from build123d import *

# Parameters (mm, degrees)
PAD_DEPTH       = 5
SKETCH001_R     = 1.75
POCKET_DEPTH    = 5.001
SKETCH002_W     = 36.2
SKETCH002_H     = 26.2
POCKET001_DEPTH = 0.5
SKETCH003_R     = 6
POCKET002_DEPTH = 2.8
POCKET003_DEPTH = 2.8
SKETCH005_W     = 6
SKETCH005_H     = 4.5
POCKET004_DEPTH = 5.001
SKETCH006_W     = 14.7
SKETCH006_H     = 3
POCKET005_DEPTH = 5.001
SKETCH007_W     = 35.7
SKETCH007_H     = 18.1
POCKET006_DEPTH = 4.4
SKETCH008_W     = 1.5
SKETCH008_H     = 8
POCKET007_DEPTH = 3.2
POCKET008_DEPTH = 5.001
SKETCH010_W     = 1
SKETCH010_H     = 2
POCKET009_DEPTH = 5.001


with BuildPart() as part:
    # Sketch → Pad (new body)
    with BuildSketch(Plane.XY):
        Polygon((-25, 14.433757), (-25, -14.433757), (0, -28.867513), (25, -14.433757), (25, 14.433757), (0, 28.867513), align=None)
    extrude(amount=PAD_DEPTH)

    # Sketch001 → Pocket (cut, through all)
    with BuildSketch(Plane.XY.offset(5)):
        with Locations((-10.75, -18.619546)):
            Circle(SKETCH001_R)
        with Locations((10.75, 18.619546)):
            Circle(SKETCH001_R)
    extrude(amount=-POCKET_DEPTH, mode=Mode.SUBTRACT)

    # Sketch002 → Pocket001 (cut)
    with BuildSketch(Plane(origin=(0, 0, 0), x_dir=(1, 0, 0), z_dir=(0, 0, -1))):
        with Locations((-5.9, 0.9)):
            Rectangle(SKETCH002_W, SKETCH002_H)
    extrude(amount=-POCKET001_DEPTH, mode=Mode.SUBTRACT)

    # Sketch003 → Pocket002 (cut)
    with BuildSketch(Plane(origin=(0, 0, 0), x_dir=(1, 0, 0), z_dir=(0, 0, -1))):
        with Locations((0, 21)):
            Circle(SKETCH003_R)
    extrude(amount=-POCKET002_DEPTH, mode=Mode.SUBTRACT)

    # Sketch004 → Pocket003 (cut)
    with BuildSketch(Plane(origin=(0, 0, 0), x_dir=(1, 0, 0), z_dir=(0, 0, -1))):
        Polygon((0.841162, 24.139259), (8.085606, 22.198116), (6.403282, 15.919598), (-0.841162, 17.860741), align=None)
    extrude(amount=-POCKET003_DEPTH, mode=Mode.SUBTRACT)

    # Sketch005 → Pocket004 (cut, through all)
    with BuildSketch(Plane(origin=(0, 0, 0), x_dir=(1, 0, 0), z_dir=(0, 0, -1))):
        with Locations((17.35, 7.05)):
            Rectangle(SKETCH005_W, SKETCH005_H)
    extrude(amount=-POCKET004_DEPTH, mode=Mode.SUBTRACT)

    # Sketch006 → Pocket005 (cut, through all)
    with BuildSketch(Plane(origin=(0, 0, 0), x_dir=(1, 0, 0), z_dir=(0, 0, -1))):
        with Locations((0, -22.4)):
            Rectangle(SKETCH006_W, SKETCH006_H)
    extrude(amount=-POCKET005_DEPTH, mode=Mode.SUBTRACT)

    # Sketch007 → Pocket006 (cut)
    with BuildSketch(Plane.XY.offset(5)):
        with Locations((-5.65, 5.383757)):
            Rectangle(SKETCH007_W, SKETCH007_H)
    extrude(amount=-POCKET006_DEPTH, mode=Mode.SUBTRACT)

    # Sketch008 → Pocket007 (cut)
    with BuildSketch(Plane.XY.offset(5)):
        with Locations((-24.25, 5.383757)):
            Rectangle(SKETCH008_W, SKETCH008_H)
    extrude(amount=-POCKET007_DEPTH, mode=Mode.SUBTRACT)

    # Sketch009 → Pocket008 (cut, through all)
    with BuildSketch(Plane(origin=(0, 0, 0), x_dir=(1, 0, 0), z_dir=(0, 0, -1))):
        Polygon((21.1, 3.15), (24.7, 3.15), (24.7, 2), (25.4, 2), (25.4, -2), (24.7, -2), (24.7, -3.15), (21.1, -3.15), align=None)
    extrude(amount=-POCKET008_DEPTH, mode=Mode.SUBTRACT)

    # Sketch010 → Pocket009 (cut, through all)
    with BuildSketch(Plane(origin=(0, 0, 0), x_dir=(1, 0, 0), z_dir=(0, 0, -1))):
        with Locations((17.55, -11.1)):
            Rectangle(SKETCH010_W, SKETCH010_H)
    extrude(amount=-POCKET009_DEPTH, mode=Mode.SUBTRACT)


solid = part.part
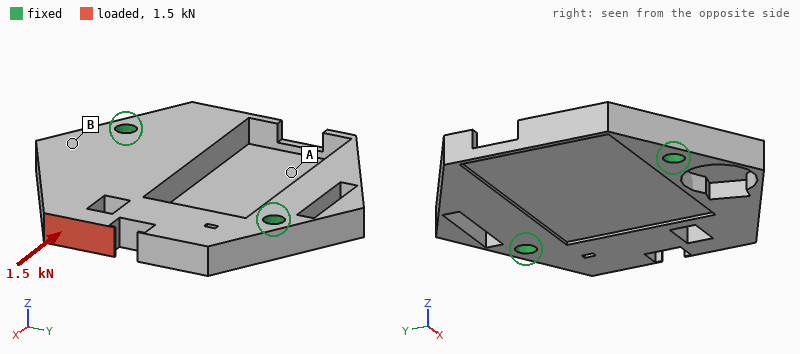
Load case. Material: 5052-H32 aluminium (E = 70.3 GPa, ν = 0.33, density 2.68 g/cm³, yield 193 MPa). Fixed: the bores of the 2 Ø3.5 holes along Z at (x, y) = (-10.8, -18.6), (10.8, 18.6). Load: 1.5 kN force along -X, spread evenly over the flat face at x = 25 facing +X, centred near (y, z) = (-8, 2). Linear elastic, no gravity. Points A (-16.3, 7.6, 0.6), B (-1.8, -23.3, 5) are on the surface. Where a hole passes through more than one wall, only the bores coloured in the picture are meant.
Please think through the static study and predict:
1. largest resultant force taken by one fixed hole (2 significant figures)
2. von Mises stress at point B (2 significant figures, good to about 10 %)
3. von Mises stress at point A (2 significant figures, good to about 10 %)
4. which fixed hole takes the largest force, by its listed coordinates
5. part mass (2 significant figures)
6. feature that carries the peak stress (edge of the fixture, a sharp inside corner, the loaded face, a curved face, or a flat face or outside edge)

1.3 kN
11 MPa
30 MPa
(-10.8, -18.6)
18 g
the loaded face
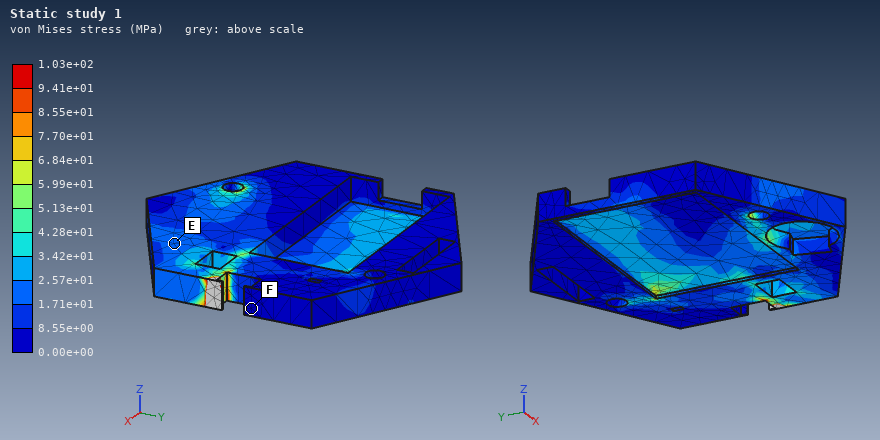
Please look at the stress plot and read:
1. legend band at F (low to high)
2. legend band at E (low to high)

0.00e+00 to 8.55e+00 MPa
1.71e+01 to 2.57e+01 MPa
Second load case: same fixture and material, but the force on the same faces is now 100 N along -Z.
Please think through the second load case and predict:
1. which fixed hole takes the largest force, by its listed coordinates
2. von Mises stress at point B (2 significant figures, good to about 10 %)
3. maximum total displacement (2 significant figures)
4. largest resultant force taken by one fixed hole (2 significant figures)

(10.8, 18.6)
14 MPa
68 µm
66 N
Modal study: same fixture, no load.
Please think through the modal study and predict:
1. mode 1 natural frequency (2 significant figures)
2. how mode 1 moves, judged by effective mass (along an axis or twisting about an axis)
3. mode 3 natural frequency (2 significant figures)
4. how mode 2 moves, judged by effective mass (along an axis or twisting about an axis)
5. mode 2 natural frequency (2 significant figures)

4400 Hz
along Z
11 kHz
along Z
5300 Hz
